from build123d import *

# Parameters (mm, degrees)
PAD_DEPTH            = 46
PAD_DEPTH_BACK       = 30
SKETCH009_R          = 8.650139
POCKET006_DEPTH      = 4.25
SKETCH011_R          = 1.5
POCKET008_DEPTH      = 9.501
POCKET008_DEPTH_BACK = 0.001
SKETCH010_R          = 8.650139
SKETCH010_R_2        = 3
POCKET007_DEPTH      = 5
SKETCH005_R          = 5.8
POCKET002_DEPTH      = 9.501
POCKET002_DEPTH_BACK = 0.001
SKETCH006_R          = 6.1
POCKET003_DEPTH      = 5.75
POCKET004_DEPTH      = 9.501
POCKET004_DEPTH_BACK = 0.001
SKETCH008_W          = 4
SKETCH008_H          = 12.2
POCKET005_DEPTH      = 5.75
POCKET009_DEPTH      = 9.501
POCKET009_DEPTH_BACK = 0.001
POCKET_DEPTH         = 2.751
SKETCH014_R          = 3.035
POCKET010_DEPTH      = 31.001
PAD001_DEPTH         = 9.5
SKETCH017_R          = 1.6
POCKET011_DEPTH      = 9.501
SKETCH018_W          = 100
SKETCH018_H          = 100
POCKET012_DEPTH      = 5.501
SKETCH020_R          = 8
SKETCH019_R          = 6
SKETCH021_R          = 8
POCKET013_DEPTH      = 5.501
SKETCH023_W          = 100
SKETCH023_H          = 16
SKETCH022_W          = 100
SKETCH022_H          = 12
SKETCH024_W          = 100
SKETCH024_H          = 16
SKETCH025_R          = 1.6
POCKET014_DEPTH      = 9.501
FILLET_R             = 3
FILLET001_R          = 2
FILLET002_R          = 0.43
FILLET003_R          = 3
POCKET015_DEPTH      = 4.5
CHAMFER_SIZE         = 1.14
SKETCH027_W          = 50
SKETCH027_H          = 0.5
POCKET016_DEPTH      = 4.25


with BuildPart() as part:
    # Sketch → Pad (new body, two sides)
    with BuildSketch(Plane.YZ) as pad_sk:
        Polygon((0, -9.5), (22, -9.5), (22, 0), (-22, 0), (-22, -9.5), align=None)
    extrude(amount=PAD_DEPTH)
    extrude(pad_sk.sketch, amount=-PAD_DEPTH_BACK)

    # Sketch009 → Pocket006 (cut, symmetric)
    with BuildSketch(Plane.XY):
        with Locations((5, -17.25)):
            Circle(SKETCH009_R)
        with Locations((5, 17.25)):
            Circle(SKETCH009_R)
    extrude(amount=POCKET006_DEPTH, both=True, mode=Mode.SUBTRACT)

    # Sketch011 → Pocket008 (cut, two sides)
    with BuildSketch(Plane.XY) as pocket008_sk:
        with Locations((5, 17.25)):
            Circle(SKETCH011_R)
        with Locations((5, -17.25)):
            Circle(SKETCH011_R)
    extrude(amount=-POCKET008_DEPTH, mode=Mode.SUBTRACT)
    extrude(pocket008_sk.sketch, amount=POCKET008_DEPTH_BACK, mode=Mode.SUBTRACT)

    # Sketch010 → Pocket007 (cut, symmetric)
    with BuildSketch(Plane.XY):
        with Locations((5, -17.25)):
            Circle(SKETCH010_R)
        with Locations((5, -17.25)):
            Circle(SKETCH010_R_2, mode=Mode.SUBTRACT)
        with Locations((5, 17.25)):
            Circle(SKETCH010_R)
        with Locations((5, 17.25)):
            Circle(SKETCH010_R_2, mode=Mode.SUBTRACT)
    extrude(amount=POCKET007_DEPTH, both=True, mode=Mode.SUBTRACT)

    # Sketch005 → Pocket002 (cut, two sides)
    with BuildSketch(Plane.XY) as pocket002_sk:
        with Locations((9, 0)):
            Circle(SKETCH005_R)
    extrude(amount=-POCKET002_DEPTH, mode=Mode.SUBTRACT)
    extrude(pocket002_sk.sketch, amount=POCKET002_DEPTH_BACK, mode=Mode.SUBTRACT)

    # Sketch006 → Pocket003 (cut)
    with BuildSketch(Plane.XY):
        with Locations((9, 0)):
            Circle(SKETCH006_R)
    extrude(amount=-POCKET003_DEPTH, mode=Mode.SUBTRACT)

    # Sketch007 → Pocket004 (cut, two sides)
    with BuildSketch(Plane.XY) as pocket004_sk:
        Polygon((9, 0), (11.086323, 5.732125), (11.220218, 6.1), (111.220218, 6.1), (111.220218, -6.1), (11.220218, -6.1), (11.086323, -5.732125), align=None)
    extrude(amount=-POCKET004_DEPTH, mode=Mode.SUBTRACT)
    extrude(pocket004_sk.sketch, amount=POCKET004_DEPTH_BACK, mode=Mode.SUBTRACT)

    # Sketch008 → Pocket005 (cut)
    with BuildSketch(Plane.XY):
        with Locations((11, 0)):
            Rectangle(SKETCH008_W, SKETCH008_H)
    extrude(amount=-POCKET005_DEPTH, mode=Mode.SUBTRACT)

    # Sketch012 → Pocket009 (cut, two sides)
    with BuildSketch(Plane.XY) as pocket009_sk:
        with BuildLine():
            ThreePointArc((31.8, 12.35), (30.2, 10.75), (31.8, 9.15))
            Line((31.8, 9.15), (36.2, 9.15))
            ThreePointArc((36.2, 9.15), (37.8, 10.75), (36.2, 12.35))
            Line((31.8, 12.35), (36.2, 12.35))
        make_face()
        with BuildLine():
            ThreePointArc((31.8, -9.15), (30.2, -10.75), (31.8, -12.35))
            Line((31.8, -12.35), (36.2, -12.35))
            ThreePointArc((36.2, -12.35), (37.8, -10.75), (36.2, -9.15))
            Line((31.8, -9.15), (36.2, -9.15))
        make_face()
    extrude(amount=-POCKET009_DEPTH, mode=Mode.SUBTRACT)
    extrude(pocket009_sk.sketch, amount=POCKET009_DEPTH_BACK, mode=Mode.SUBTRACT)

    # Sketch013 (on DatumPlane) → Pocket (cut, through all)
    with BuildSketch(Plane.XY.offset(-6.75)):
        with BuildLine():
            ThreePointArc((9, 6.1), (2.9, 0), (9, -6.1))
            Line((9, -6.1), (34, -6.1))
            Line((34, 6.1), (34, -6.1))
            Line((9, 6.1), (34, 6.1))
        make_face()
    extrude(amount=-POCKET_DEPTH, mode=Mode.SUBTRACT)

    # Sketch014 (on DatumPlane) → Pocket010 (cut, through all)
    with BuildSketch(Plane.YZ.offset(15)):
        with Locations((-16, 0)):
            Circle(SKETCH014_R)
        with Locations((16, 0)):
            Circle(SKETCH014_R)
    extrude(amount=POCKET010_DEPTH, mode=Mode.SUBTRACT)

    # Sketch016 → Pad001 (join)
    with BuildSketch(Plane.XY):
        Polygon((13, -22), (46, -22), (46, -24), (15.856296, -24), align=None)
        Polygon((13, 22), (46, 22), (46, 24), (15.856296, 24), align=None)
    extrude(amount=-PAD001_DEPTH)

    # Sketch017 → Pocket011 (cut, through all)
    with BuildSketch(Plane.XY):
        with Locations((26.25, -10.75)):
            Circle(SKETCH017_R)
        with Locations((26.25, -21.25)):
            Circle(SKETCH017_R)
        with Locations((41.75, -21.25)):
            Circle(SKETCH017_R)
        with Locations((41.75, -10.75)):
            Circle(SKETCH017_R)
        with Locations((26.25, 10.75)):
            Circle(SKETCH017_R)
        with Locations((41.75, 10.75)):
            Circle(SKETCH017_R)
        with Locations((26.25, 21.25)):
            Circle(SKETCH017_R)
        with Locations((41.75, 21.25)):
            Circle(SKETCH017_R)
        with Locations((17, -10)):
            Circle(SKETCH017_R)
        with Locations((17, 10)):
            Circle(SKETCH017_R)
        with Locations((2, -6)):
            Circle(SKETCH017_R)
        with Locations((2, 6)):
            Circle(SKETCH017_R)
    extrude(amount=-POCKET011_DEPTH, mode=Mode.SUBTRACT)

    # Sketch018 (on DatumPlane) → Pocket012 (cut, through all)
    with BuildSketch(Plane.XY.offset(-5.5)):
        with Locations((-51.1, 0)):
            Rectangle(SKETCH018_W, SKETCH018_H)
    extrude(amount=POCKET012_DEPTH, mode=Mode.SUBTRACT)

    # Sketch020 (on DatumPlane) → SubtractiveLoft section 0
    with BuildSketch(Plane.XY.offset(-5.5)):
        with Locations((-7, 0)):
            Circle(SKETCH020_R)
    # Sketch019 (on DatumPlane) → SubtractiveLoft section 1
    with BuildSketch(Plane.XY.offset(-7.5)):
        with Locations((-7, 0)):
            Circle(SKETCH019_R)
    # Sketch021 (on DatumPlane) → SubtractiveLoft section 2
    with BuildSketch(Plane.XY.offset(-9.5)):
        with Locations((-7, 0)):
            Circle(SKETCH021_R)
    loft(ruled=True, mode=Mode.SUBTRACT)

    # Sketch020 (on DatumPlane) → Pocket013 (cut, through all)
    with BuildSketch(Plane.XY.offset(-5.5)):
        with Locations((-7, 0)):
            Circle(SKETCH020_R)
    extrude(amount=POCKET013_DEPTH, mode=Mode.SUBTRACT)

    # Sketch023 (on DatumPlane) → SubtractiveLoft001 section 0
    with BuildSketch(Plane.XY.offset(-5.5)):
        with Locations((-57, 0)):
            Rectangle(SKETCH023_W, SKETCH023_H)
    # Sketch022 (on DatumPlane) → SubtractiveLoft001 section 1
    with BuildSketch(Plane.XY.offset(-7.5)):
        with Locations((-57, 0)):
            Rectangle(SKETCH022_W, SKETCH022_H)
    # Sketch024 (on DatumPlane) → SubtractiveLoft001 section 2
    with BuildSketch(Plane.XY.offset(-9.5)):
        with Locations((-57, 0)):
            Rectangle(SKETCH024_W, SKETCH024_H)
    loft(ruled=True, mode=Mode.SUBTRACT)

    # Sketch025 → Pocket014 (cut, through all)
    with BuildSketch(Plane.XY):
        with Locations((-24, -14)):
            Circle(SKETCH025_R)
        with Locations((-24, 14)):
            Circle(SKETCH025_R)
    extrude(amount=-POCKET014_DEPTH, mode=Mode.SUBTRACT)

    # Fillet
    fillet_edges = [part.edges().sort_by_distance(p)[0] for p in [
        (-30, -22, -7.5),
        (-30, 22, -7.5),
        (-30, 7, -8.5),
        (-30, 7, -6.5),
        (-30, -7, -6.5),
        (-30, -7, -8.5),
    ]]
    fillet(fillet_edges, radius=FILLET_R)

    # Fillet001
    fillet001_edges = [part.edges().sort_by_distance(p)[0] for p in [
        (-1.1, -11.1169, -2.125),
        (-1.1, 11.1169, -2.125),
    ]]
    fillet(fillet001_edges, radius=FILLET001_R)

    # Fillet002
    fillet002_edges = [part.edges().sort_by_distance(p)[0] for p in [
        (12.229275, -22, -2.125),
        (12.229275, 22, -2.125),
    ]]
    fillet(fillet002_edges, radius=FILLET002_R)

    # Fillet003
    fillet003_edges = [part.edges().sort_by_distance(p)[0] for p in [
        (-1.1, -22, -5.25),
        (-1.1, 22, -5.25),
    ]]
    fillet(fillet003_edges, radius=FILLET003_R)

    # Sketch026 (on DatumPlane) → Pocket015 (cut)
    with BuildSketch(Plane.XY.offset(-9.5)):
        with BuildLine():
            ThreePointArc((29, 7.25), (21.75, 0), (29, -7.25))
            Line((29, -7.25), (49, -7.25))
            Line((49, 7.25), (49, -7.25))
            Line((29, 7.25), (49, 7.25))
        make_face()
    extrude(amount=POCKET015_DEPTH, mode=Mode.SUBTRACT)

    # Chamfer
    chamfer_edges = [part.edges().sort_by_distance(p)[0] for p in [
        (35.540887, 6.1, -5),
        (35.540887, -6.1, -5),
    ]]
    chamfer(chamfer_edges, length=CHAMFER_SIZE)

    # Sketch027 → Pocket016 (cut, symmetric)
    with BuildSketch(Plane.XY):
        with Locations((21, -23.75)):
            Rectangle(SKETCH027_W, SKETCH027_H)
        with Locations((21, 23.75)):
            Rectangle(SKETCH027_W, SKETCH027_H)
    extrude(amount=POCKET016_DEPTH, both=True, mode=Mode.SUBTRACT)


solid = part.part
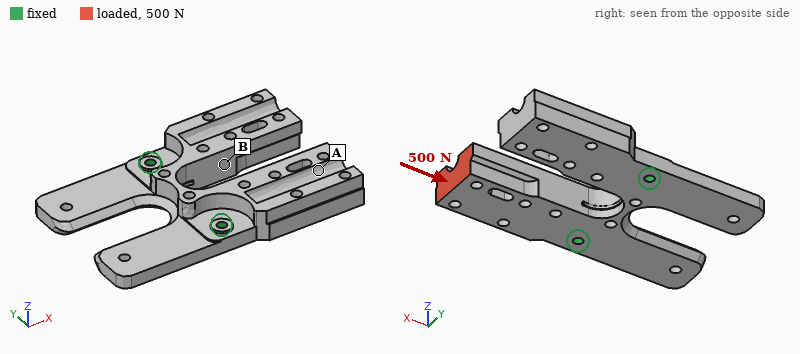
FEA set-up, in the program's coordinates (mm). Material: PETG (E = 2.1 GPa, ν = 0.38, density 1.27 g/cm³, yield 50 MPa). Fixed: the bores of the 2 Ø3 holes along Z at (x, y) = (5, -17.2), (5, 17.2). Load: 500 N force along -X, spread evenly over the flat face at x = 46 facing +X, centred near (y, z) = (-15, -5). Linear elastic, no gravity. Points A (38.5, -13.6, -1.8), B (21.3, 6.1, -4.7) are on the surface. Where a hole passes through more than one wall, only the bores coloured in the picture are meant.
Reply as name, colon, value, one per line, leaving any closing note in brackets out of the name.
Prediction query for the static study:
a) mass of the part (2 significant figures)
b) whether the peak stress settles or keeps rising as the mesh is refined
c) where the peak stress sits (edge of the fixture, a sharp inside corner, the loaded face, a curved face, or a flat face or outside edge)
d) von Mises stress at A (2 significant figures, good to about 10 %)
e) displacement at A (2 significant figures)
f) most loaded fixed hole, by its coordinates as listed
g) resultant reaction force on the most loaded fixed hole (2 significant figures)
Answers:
mass of the part: 19 g
whether the peak stress settles or keeps rising as the mesh is refined: keeps rising
where the peak stress sits: edge of the fixture
von Mises stress at A: 6.3 MPa
displacement at A: 0.80 mm
most loaded fixed hole, by its coordinates as listed: (5, -17.2)
resultant reaction force on the most loaded fixed hole: 470 N
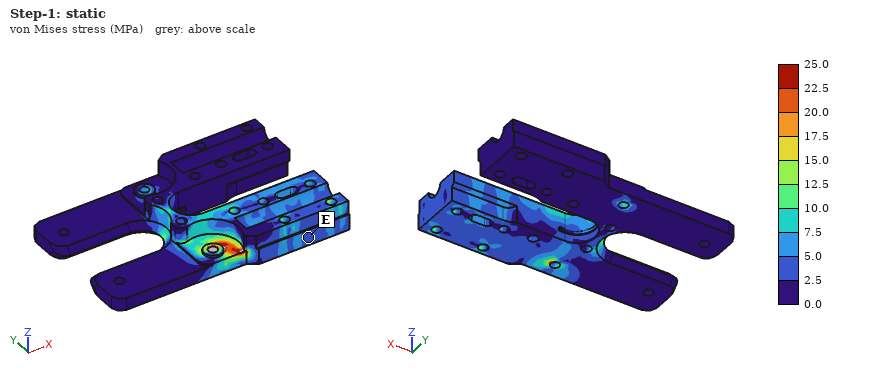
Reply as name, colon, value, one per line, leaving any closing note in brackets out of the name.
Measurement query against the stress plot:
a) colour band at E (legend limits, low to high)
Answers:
colour band at E: 2.5 to 5.0 MPa
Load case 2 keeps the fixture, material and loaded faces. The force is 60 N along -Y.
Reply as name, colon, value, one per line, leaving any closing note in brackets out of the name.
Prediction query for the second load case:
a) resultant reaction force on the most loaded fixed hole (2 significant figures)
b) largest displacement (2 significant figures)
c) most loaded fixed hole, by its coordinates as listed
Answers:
resultant reaction force on the most loaded fixed hole: 140 N
largest displacement: 0.88 mm
most loaded fixed hole, by its coordinates as listed: (5, -17.2)
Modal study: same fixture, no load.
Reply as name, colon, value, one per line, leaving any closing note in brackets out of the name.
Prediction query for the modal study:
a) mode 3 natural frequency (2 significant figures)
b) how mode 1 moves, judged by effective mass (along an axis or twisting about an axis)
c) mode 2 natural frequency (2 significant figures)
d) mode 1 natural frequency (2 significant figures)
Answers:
mode 3 natural frequency: 770 Hz
how mode 1 moves, judged by effective mass: along Z
mode 2 natural frequency: 570 Hz
mode 1 natural frequency: 530 Hz
